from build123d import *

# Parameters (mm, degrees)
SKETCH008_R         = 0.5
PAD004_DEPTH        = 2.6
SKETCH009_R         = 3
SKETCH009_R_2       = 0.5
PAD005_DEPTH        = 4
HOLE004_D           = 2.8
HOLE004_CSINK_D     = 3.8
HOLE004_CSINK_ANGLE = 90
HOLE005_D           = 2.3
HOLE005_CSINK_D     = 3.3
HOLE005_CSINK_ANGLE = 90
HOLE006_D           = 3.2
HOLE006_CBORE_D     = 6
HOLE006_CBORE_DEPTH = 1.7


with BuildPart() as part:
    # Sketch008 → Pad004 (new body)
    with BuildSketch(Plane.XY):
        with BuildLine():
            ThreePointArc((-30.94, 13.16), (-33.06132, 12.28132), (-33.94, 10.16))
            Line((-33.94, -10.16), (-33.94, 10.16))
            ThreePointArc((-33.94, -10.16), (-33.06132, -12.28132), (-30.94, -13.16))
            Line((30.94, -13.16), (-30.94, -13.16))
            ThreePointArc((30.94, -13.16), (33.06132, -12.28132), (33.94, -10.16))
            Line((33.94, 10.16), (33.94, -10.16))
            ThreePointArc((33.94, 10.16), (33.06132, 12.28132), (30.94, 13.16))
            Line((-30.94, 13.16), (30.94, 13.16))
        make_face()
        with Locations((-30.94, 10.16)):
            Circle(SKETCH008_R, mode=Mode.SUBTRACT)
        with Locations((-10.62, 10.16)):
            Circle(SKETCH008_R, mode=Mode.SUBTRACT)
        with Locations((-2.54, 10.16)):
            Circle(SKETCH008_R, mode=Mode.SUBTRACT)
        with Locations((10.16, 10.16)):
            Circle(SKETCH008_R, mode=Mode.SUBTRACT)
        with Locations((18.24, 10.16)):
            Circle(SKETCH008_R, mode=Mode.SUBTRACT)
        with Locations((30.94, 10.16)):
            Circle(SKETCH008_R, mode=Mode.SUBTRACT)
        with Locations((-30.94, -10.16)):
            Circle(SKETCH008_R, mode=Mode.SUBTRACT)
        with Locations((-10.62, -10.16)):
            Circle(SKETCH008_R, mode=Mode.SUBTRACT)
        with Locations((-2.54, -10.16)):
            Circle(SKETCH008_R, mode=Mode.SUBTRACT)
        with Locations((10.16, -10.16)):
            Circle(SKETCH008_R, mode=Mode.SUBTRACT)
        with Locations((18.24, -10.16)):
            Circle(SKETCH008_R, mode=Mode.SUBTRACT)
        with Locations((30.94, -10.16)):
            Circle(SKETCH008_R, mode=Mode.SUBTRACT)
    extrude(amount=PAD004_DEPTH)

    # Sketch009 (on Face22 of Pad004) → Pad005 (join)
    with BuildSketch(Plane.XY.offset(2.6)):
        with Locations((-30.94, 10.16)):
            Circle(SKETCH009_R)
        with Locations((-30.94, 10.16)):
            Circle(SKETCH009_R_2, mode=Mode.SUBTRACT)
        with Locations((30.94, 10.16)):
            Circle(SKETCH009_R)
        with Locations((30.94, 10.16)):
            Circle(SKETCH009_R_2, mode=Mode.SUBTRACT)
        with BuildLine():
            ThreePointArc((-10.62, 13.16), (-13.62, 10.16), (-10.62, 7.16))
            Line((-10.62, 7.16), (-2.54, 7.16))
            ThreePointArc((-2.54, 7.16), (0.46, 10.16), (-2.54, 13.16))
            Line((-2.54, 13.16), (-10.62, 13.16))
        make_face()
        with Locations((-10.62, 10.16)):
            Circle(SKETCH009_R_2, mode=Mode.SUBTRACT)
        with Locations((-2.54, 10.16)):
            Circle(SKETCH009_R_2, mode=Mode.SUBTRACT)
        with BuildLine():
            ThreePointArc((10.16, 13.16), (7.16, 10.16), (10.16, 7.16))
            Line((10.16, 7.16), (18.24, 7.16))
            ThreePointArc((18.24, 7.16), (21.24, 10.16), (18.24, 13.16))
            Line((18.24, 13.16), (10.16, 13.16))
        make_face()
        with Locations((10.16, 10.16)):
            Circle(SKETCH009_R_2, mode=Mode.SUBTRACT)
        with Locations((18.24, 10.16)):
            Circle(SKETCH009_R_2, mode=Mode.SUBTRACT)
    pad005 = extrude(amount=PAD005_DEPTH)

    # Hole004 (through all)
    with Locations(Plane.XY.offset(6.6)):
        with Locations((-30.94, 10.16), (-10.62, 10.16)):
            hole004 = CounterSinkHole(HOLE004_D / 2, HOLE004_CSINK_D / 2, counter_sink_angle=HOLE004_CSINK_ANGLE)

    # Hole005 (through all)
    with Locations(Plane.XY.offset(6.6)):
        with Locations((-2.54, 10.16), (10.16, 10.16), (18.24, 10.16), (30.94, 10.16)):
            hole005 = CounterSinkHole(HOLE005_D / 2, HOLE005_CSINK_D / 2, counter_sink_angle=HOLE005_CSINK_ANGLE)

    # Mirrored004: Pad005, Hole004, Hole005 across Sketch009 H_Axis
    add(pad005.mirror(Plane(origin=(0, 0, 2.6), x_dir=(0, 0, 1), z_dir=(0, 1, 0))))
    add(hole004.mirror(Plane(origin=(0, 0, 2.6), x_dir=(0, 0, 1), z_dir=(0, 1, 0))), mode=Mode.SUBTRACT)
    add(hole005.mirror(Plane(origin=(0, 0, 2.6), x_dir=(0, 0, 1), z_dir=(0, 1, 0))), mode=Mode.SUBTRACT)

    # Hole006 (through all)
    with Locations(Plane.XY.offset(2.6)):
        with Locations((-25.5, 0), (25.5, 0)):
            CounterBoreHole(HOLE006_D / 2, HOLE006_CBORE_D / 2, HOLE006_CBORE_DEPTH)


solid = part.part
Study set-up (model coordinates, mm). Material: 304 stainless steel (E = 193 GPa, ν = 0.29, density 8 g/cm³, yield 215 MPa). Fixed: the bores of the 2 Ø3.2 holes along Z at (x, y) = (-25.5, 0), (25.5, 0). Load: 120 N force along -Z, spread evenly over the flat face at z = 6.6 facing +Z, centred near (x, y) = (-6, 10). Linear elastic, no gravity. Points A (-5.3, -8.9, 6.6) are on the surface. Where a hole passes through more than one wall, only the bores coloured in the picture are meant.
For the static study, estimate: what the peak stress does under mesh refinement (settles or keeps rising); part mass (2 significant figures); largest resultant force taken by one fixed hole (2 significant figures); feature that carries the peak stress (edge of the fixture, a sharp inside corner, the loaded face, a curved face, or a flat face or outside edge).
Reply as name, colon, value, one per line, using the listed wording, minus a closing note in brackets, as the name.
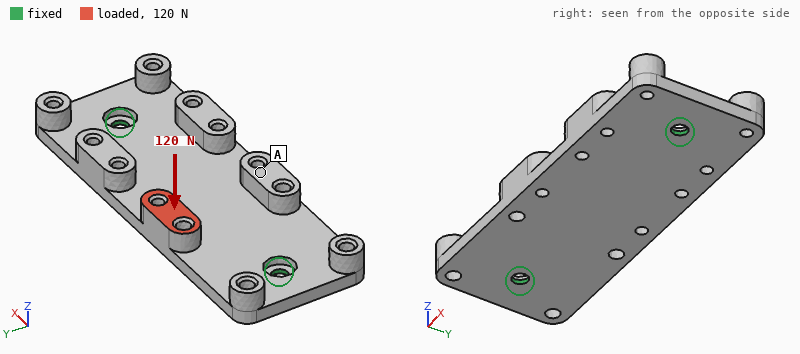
what the peak stress does under mesh refinement: keeps rising
part mass: 46 g
largest resultant force taken by one fixed hole: 190 N
feature that carries the peak stress: edge of the fixture
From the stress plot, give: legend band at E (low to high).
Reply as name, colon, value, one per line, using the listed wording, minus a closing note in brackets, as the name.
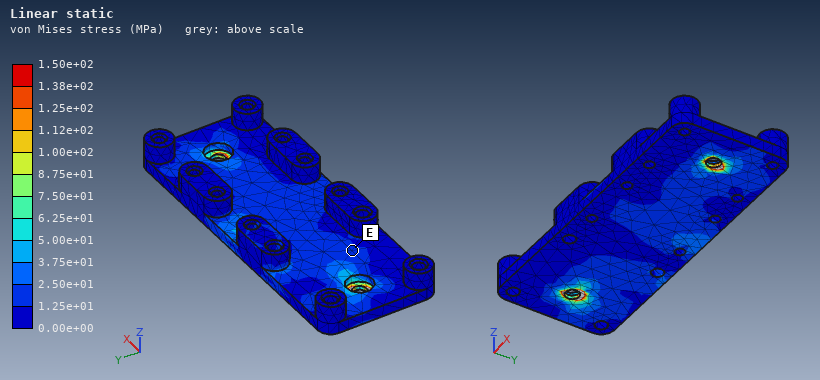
legend band at E: 1.25e+01 to 2.50e+01 MPa
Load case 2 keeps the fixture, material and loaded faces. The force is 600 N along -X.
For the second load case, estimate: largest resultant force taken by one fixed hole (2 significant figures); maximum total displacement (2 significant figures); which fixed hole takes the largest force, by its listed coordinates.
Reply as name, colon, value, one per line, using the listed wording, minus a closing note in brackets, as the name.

largest resultant force taken by one fixed hole: 390 N
maximum total displacement: 25 µm
which fixed hole takes the largest force, by its listed coordinates: (25.5, 0)
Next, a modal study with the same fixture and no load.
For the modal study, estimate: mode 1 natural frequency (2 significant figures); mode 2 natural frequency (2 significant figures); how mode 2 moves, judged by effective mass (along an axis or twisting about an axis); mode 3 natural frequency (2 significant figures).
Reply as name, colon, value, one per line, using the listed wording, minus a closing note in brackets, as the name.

mode 1 natural frequency: 2500 Hz
mode 2 natural frequency: 3300 Hz
how mode 2 moves, judged by effective mass: along Z
mode 3 natural frequency: 5700 Hz
